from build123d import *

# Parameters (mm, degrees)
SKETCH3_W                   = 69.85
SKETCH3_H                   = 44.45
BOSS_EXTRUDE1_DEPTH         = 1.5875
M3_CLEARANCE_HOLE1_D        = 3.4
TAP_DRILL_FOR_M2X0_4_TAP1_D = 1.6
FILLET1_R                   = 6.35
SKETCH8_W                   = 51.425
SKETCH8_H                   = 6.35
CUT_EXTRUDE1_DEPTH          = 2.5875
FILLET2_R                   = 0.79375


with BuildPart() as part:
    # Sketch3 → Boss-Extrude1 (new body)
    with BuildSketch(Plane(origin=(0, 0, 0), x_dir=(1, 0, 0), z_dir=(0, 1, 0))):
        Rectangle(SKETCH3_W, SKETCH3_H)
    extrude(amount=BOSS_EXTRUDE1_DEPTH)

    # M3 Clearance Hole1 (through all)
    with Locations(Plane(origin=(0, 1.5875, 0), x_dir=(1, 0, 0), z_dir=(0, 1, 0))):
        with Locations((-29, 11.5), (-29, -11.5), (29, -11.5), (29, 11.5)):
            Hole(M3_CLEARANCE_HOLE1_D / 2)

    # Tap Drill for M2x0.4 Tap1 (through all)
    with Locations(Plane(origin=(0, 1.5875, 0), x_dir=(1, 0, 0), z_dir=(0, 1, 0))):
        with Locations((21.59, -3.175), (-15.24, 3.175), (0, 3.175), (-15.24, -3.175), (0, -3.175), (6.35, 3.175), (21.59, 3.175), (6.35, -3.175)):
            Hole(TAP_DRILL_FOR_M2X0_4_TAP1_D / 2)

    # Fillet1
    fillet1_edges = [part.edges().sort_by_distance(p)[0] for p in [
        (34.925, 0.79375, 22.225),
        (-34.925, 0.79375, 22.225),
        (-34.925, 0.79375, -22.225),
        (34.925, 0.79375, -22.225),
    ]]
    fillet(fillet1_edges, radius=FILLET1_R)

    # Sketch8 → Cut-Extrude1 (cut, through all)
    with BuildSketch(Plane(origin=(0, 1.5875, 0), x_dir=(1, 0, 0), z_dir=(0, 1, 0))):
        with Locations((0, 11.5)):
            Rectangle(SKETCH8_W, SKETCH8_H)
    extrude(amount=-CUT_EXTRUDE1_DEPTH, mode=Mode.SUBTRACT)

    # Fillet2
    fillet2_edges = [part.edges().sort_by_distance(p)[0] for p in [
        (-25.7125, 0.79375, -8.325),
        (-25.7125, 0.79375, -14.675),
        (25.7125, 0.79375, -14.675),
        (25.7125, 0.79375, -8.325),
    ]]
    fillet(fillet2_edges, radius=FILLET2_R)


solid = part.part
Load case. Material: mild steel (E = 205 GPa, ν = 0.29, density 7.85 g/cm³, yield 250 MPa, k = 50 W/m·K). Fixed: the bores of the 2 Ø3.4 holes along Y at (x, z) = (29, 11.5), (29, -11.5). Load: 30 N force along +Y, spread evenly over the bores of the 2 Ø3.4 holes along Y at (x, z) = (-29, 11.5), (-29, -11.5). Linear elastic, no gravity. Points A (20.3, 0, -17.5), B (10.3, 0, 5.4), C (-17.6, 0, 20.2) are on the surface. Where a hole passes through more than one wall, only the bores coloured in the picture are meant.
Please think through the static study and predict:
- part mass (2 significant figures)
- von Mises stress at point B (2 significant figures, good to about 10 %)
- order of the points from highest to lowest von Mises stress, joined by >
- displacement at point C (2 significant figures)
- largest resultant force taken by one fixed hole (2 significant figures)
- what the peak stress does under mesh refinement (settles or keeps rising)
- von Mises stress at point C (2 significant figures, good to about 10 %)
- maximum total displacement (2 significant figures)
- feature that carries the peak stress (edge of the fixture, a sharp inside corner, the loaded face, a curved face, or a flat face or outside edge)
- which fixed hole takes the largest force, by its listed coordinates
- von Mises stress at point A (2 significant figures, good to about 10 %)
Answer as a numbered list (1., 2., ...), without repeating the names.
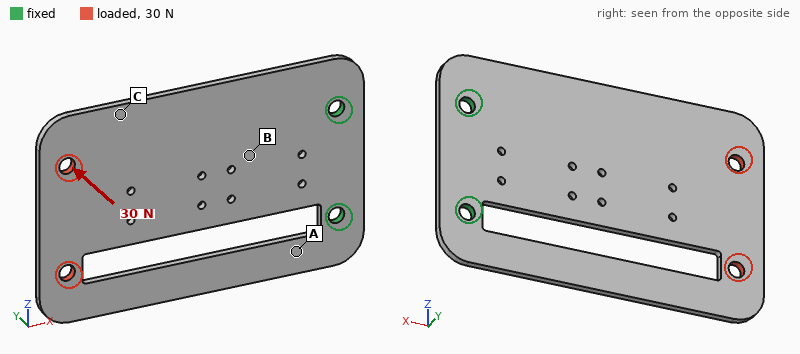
1. 34 g
2. 68 MPa
3. A > B > C
4. 0.53 mm
5. 26 N
6. keeps rising
7. 22 MPa
8. 0.91 mm
9. edge of the fixture
10. (29, 11.5)
11. 94 MPa
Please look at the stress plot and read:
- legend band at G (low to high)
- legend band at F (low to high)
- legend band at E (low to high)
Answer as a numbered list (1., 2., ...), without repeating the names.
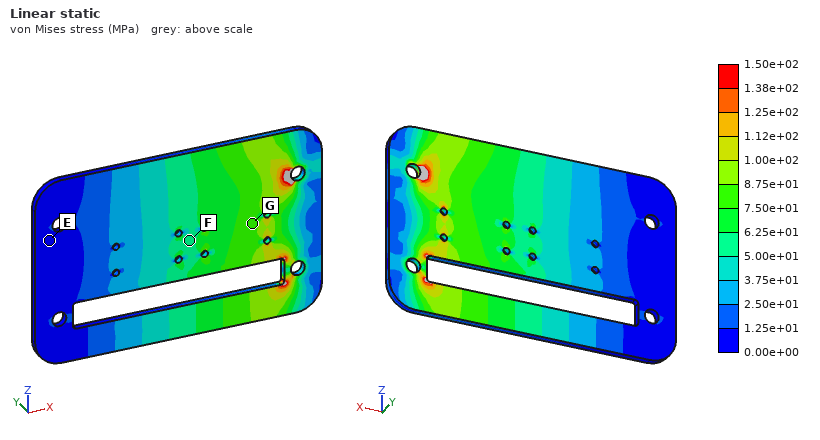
1. 7.50e+01 to 8.75e+01 MPa
2. 5.00e+01 to 6.25e+01 MPa
3. 0.00e+00 to 1.25e+01 MPa
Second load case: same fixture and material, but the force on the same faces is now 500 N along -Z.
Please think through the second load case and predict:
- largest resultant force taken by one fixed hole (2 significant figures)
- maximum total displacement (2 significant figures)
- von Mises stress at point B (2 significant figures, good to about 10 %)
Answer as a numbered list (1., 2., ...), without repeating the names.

1. 1.2 kN
2. 62 µm
3. 28 MPa
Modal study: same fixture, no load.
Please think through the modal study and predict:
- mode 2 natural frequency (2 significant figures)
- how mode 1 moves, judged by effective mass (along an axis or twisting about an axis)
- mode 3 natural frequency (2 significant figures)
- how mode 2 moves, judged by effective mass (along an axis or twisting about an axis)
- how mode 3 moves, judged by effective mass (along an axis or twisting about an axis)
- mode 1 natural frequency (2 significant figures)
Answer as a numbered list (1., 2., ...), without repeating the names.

1. 990 Hz
2. along Y
3. 1900 Hz
4. twisting about X
5. along Y
6. 310 Hz
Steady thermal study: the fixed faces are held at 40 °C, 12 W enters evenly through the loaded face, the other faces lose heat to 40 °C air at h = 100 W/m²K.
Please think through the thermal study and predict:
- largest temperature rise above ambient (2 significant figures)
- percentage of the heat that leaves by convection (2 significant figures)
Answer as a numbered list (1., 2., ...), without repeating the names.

1. 75 K
2. 94 %
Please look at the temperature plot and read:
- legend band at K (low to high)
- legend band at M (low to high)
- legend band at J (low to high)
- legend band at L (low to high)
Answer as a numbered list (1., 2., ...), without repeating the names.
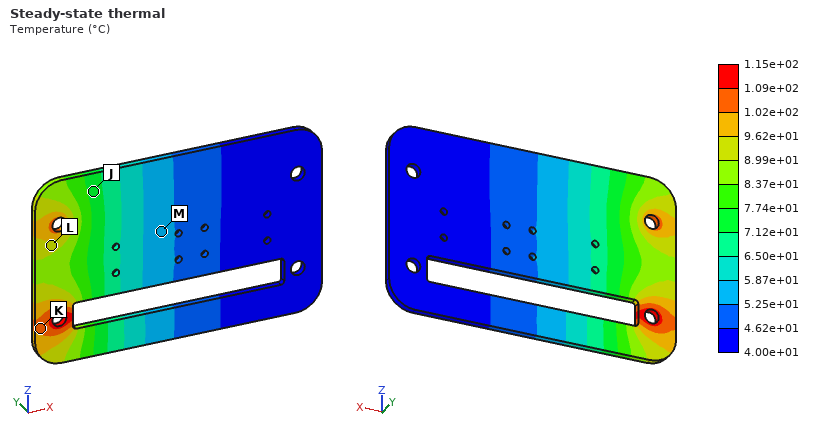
1. 1.02e+02 to 1.09e+02 °C
2. 5.25e+01 to 5.87e+01 °C
3. 7.12e+01 to 7.74e+01 °C
4. 8.99e+01 to 9.62e+01 °C
